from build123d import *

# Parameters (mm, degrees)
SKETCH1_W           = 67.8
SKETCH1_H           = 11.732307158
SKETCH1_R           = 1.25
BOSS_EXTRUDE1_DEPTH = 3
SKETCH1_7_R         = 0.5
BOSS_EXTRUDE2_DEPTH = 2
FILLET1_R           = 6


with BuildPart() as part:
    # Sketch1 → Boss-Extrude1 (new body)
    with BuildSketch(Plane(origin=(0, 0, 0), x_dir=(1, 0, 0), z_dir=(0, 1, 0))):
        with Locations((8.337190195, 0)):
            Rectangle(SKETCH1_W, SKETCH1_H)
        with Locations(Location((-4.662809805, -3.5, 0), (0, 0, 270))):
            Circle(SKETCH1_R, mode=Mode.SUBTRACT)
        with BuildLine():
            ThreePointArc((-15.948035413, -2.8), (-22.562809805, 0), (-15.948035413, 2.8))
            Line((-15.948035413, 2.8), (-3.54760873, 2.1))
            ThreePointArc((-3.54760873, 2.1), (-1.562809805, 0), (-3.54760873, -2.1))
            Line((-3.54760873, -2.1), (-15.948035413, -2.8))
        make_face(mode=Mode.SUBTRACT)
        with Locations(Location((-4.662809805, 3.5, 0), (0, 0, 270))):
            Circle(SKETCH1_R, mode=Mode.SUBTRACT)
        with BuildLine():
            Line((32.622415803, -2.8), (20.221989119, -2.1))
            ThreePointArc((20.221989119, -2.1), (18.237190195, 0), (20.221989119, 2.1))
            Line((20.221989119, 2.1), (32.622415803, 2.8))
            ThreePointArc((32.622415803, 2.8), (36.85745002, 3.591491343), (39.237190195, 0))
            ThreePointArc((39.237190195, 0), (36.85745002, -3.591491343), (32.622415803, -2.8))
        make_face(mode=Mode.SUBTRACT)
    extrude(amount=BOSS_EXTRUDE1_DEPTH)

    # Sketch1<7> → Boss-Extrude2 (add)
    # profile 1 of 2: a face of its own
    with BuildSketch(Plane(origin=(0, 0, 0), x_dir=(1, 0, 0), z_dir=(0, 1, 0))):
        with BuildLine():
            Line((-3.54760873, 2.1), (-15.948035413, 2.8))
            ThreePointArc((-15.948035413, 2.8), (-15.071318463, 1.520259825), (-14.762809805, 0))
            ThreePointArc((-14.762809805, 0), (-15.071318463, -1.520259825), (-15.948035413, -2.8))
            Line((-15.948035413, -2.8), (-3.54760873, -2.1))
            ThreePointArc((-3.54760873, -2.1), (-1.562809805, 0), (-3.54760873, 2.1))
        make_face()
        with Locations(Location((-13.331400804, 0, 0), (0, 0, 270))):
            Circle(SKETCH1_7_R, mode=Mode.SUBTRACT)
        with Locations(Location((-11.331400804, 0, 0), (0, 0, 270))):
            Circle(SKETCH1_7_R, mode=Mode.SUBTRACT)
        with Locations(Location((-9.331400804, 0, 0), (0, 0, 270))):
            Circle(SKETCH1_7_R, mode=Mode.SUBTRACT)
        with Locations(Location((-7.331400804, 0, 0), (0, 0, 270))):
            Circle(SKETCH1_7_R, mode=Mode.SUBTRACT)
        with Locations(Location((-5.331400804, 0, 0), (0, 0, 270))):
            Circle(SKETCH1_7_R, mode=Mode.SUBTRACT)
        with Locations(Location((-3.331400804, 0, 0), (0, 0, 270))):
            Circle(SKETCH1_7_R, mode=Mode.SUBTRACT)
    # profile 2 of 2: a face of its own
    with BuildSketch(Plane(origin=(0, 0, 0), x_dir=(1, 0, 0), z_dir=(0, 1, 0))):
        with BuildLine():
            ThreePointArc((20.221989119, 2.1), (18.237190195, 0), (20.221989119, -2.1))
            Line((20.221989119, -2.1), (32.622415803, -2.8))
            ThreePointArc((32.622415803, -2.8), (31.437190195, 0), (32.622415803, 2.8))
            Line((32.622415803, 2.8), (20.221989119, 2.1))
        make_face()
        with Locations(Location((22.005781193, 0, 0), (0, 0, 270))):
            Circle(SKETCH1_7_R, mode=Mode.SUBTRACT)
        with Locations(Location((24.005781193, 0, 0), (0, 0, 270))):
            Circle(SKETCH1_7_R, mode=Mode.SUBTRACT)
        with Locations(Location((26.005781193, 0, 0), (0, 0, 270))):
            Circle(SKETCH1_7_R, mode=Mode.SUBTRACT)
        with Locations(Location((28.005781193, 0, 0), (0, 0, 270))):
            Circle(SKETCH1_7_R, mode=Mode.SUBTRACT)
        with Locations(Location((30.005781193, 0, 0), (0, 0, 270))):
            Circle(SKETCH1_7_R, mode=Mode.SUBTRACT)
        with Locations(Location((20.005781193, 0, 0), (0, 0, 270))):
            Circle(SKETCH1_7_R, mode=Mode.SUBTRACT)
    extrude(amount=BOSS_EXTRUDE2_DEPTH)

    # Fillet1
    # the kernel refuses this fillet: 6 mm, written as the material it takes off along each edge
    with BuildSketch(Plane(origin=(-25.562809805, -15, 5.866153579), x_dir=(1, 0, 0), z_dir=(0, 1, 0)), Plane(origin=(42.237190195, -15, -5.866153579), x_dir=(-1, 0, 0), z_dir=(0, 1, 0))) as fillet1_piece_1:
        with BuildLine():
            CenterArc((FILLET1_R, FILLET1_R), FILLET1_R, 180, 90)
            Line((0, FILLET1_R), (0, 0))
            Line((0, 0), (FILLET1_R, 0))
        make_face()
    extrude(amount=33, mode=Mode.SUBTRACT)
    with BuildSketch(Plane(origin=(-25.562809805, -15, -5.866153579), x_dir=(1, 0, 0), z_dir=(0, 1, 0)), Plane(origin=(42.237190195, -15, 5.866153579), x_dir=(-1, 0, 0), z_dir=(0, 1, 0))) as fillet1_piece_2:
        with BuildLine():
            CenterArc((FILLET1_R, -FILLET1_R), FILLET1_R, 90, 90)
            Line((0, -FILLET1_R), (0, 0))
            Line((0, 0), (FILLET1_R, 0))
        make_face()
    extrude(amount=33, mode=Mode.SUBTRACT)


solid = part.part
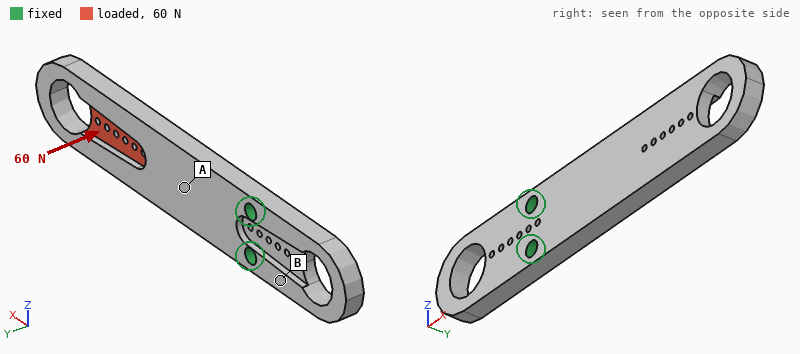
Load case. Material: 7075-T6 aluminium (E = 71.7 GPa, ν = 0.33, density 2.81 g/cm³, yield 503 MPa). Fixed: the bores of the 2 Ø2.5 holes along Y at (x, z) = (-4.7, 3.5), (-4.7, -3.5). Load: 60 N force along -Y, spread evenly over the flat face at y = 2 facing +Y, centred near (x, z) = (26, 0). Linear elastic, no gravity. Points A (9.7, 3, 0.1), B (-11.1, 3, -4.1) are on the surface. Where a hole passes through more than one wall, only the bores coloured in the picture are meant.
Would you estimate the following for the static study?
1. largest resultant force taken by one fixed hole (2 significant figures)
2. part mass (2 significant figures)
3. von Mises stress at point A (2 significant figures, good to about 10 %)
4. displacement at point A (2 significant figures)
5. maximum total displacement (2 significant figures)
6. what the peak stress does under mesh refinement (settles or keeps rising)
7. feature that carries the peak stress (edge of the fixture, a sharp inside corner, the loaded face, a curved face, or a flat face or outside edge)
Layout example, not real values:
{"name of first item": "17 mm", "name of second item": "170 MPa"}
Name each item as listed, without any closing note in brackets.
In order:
{"largest resultant force taken by one fixed hole": "30 N", "part mass": "5.2 g", "von Mises stress at point A": "54 MPa", "displacement at point A": "0.083 mm", "maximum total displacement": "0.54 mm", "what the peak stress does under mesh refinement": "keeps rising", "feature that carries the peak stress": "edge of the fixture"}
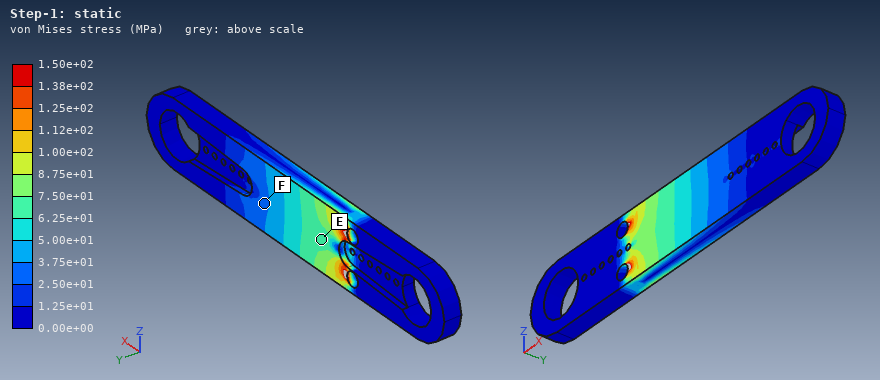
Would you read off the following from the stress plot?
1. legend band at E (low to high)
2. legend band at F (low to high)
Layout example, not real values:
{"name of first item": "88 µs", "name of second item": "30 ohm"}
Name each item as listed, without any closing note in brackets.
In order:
{"legend band at E": "6.25e+01 to 7.50e+01 MPa", "legend band at F": "2.50e+01 to 3.75e+01 MPa"}
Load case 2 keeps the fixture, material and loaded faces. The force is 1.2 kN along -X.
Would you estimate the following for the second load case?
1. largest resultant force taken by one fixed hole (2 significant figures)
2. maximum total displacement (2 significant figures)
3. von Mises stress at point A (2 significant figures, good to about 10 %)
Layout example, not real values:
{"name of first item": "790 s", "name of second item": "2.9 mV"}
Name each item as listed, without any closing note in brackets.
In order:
{"largest resultant force taken by one fixed hole": "610 N", "maximum total displacement": "0.34 mm", "von Mises stress at point A": "67 MPa"}
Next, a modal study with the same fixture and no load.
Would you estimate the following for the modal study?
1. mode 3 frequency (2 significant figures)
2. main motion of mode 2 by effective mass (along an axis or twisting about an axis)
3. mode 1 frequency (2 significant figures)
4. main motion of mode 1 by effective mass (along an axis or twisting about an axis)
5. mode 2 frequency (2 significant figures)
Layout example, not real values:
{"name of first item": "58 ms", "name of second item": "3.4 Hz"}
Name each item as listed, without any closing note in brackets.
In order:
{"mode 3 frequency": "6800 Hz", "main motion of mode 2 by effective mass": "along Z", "mode 1 frequency": "1400 Hz", "main motion of mode 1 by effective mass": "along Y", "mode 2 frequency": "5200 Hz"}
